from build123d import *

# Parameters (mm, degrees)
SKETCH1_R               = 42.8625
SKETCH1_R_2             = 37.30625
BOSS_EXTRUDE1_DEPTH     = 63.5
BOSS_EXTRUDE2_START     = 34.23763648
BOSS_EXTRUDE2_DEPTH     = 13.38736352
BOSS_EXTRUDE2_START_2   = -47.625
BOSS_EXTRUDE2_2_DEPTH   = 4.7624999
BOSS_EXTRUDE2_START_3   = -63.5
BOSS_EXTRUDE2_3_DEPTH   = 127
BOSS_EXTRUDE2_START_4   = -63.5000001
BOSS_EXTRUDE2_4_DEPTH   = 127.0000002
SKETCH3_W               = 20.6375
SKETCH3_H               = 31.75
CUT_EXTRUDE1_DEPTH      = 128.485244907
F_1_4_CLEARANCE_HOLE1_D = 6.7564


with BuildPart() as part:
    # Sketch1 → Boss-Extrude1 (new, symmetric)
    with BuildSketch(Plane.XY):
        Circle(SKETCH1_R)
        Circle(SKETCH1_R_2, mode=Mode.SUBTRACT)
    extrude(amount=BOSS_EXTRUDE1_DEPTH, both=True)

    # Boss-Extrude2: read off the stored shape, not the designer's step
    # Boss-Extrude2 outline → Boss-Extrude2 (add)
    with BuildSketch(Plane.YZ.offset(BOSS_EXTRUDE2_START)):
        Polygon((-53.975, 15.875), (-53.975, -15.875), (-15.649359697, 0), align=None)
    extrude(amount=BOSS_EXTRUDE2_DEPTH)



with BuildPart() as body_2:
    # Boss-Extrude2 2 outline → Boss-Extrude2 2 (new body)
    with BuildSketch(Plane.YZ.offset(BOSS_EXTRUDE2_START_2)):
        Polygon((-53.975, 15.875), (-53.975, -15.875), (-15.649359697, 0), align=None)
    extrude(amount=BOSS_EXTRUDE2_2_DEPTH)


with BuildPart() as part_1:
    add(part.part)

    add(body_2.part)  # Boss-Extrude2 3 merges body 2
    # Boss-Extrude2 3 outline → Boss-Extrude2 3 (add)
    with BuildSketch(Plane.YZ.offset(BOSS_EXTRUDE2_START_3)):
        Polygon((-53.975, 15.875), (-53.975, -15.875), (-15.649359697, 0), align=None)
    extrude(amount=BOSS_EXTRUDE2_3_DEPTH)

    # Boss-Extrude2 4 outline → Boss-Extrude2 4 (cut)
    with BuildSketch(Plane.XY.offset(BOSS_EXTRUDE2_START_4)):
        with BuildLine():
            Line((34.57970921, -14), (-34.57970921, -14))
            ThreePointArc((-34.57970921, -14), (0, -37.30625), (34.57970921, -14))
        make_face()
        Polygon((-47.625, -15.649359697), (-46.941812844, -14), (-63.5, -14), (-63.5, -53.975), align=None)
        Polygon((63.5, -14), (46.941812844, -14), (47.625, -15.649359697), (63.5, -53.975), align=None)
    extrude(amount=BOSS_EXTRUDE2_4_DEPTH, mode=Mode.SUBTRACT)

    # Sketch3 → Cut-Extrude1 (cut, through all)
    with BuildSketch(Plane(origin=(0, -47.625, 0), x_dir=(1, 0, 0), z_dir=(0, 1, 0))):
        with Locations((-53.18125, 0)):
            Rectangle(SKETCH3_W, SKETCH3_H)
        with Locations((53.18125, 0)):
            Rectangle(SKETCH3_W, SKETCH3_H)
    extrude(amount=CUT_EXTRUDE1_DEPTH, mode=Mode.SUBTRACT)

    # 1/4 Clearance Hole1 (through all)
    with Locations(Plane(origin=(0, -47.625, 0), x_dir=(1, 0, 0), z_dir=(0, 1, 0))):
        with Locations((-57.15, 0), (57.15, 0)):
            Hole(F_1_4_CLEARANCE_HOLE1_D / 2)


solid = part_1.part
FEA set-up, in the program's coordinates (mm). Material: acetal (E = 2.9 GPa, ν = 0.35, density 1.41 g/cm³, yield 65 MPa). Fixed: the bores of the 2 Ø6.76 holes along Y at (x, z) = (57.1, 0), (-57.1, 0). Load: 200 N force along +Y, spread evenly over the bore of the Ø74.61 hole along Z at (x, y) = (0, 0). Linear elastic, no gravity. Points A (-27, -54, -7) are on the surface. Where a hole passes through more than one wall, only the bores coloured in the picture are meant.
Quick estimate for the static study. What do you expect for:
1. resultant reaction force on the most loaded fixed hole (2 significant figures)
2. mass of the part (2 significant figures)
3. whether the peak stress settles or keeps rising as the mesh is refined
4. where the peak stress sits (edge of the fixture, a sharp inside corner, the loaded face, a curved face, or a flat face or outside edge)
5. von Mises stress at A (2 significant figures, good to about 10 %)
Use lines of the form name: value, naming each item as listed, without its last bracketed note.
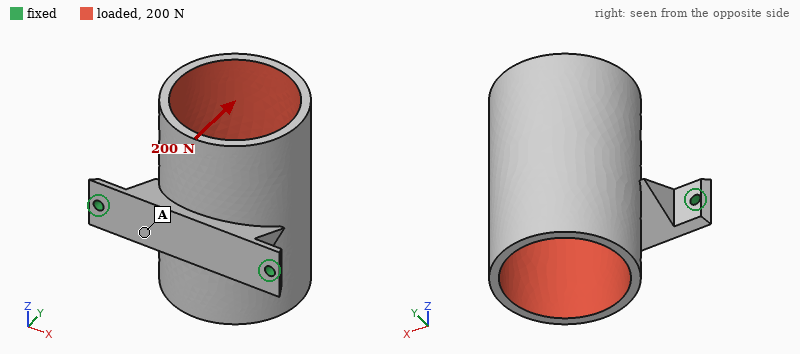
resultant reaction force on the most loaded fixed hole: 120 N
mass of the part: 310 g
whether the peak stress settles or keeps rising as the mesh is refined: keeps rising
where the peak stress sits: edge of the fixture
von Mises stress at A: 0.38 MPa
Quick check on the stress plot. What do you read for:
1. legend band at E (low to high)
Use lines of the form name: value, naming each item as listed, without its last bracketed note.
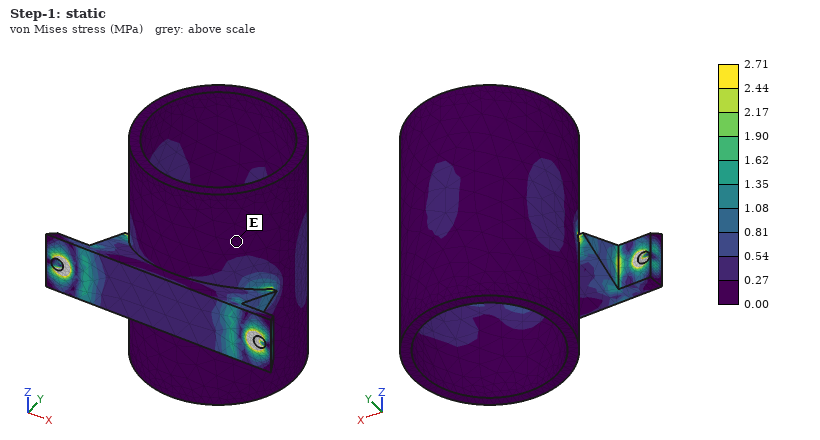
legend band at E: 0.00 to 0.27 MPa
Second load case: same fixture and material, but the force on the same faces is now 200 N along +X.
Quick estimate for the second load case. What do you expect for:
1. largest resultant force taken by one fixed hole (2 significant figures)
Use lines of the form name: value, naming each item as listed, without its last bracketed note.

largest resultant force taken by one fixed hole: 140 N
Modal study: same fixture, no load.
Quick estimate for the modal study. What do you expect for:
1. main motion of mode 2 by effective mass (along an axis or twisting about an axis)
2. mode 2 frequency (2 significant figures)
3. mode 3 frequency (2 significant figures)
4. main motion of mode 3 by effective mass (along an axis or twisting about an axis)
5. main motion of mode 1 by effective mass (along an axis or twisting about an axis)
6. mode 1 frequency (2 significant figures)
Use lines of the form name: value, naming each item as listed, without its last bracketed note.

main motion of mode 2 by effective mass: along X
mode 2 frequency: 280 Hz
mode 3 frequency: 430 Hz
main motion of mode 3 by effective mass: twisting about Y
main motion of mode 1 by effective mass: along Z
mode 1 frequency: 84 Hz
